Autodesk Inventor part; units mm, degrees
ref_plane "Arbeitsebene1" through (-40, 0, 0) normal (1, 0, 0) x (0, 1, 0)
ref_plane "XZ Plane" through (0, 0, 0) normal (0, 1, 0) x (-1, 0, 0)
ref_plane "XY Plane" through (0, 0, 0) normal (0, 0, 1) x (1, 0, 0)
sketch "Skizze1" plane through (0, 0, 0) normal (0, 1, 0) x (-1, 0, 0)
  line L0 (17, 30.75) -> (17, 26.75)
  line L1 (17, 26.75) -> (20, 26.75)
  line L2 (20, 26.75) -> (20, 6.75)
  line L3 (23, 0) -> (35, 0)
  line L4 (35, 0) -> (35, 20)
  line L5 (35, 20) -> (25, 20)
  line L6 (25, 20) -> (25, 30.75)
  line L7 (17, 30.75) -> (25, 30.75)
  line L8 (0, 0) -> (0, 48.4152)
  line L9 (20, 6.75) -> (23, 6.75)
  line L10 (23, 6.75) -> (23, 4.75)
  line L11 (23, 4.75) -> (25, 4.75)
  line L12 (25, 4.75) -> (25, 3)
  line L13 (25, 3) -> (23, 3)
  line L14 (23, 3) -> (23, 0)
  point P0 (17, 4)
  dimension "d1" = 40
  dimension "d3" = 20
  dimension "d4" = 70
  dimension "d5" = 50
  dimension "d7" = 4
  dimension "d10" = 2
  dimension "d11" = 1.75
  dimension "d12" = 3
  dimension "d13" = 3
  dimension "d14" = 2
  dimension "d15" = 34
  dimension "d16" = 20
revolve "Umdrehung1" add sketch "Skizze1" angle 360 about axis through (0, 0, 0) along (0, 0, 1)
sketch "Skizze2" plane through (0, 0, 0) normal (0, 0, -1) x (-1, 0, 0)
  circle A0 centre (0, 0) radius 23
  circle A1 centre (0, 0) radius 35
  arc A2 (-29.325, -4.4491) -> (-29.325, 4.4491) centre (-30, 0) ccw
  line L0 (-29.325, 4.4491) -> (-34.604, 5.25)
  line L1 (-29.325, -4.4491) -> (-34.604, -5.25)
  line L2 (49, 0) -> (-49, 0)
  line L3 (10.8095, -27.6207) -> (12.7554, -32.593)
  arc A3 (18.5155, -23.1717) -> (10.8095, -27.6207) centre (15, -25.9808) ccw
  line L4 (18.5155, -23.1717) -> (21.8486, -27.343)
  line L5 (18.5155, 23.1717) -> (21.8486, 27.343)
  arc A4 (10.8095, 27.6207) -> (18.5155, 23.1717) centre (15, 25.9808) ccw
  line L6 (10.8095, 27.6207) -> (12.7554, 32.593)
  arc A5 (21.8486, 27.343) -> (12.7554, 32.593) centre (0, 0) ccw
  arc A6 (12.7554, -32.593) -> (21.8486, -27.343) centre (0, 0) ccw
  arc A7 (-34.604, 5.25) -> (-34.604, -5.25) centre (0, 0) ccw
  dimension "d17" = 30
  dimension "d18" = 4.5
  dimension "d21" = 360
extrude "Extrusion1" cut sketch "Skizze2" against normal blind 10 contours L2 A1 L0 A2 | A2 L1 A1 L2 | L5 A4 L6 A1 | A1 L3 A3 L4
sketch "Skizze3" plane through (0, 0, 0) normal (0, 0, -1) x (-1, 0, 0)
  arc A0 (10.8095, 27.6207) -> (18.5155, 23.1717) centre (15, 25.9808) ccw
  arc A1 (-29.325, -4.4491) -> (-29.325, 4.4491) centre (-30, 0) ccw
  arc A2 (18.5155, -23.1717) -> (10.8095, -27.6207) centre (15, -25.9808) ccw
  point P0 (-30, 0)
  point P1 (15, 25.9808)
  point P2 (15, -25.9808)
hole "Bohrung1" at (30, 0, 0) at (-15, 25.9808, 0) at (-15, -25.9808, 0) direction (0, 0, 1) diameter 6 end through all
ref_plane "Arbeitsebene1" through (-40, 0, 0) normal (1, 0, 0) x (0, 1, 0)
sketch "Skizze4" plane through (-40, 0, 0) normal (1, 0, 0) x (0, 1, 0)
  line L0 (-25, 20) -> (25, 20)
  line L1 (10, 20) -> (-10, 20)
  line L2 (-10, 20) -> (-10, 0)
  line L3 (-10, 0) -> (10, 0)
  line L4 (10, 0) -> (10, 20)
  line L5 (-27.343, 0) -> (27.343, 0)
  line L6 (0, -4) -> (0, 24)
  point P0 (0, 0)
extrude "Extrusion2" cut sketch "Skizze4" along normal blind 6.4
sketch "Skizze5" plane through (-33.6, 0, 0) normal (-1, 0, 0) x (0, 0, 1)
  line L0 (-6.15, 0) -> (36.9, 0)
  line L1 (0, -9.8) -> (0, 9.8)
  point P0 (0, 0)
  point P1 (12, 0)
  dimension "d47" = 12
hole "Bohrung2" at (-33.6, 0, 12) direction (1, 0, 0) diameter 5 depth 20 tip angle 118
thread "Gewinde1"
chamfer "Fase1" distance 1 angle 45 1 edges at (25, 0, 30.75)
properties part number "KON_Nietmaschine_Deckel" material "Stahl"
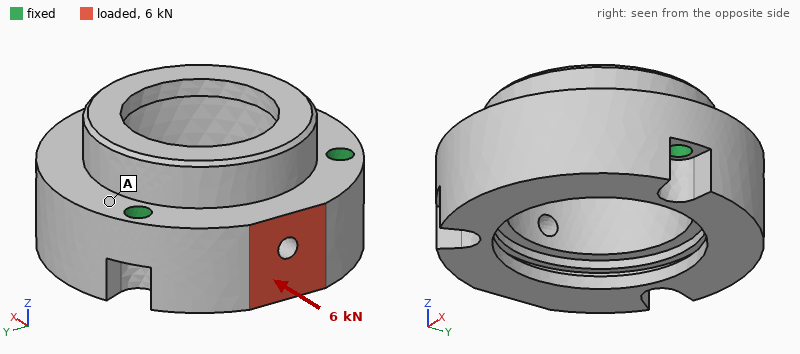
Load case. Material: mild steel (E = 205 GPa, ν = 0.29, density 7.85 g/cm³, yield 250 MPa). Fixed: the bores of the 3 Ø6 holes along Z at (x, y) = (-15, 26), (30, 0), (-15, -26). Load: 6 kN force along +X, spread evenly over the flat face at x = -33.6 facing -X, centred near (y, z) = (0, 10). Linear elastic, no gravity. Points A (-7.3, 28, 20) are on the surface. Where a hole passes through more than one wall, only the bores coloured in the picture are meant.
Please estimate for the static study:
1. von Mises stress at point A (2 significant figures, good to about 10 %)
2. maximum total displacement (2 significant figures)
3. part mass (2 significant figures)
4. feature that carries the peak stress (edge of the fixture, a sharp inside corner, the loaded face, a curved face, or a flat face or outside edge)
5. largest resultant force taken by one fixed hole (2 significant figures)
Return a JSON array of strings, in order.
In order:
["9.3 MPa", "11 µm", "420 g", "edge of the fixture", "3.9 kN"]
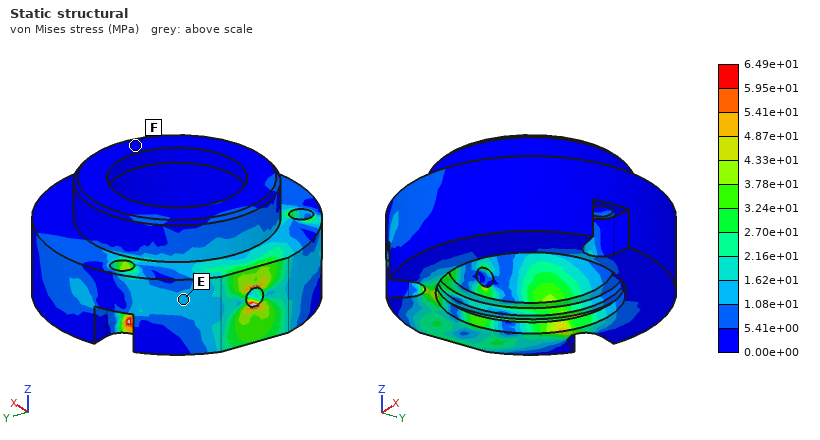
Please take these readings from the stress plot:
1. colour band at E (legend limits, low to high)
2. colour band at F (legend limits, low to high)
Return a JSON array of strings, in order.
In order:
["1.08e+01 to 1.62e+01 MPa", "0.00e+00 to 5.41e+00 MPa"]
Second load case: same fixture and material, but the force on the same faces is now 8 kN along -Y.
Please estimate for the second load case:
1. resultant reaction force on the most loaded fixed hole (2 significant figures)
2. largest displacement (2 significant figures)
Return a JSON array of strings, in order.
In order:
["4.9 kN", "5.0 µm"]
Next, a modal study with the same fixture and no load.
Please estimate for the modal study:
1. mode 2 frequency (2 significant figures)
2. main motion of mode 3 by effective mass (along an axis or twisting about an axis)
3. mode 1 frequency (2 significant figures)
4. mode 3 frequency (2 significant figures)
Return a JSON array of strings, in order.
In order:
["11 kHz", "along Z", "11 kHz", "16 kHz"]
